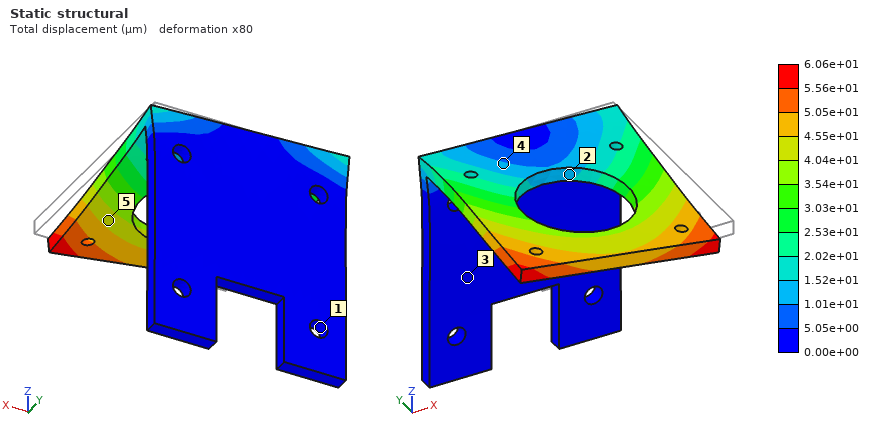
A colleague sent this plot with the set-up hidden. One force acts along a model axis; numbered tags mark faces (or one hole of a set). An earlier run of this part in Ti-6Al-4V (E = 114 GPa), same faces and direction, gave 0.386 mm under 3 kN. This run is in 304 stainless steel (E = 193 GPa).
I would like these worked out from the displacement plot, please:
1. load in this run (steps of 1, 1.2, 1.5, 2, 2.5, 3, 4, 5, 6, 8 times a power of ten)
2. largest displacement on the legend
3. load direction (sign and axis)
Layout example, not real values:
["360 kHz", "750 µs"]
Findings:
["800 N", "6.06e+01 µm", "-X"]
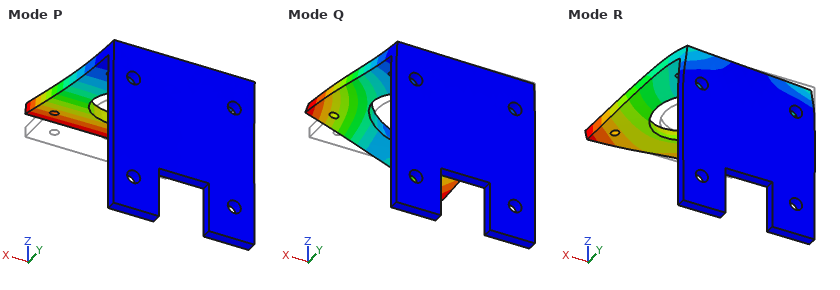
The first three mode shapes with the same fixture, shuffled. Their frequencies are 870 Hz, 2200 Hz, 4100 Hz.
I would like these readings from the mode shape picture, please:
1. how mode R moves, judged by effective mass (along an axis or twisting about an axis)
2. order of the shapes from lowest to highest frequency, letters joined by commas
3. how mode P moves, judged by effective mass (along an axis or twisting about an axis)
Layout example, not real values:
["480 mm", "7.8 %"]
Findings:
["along X", "P, Q, R", "along Z"]
